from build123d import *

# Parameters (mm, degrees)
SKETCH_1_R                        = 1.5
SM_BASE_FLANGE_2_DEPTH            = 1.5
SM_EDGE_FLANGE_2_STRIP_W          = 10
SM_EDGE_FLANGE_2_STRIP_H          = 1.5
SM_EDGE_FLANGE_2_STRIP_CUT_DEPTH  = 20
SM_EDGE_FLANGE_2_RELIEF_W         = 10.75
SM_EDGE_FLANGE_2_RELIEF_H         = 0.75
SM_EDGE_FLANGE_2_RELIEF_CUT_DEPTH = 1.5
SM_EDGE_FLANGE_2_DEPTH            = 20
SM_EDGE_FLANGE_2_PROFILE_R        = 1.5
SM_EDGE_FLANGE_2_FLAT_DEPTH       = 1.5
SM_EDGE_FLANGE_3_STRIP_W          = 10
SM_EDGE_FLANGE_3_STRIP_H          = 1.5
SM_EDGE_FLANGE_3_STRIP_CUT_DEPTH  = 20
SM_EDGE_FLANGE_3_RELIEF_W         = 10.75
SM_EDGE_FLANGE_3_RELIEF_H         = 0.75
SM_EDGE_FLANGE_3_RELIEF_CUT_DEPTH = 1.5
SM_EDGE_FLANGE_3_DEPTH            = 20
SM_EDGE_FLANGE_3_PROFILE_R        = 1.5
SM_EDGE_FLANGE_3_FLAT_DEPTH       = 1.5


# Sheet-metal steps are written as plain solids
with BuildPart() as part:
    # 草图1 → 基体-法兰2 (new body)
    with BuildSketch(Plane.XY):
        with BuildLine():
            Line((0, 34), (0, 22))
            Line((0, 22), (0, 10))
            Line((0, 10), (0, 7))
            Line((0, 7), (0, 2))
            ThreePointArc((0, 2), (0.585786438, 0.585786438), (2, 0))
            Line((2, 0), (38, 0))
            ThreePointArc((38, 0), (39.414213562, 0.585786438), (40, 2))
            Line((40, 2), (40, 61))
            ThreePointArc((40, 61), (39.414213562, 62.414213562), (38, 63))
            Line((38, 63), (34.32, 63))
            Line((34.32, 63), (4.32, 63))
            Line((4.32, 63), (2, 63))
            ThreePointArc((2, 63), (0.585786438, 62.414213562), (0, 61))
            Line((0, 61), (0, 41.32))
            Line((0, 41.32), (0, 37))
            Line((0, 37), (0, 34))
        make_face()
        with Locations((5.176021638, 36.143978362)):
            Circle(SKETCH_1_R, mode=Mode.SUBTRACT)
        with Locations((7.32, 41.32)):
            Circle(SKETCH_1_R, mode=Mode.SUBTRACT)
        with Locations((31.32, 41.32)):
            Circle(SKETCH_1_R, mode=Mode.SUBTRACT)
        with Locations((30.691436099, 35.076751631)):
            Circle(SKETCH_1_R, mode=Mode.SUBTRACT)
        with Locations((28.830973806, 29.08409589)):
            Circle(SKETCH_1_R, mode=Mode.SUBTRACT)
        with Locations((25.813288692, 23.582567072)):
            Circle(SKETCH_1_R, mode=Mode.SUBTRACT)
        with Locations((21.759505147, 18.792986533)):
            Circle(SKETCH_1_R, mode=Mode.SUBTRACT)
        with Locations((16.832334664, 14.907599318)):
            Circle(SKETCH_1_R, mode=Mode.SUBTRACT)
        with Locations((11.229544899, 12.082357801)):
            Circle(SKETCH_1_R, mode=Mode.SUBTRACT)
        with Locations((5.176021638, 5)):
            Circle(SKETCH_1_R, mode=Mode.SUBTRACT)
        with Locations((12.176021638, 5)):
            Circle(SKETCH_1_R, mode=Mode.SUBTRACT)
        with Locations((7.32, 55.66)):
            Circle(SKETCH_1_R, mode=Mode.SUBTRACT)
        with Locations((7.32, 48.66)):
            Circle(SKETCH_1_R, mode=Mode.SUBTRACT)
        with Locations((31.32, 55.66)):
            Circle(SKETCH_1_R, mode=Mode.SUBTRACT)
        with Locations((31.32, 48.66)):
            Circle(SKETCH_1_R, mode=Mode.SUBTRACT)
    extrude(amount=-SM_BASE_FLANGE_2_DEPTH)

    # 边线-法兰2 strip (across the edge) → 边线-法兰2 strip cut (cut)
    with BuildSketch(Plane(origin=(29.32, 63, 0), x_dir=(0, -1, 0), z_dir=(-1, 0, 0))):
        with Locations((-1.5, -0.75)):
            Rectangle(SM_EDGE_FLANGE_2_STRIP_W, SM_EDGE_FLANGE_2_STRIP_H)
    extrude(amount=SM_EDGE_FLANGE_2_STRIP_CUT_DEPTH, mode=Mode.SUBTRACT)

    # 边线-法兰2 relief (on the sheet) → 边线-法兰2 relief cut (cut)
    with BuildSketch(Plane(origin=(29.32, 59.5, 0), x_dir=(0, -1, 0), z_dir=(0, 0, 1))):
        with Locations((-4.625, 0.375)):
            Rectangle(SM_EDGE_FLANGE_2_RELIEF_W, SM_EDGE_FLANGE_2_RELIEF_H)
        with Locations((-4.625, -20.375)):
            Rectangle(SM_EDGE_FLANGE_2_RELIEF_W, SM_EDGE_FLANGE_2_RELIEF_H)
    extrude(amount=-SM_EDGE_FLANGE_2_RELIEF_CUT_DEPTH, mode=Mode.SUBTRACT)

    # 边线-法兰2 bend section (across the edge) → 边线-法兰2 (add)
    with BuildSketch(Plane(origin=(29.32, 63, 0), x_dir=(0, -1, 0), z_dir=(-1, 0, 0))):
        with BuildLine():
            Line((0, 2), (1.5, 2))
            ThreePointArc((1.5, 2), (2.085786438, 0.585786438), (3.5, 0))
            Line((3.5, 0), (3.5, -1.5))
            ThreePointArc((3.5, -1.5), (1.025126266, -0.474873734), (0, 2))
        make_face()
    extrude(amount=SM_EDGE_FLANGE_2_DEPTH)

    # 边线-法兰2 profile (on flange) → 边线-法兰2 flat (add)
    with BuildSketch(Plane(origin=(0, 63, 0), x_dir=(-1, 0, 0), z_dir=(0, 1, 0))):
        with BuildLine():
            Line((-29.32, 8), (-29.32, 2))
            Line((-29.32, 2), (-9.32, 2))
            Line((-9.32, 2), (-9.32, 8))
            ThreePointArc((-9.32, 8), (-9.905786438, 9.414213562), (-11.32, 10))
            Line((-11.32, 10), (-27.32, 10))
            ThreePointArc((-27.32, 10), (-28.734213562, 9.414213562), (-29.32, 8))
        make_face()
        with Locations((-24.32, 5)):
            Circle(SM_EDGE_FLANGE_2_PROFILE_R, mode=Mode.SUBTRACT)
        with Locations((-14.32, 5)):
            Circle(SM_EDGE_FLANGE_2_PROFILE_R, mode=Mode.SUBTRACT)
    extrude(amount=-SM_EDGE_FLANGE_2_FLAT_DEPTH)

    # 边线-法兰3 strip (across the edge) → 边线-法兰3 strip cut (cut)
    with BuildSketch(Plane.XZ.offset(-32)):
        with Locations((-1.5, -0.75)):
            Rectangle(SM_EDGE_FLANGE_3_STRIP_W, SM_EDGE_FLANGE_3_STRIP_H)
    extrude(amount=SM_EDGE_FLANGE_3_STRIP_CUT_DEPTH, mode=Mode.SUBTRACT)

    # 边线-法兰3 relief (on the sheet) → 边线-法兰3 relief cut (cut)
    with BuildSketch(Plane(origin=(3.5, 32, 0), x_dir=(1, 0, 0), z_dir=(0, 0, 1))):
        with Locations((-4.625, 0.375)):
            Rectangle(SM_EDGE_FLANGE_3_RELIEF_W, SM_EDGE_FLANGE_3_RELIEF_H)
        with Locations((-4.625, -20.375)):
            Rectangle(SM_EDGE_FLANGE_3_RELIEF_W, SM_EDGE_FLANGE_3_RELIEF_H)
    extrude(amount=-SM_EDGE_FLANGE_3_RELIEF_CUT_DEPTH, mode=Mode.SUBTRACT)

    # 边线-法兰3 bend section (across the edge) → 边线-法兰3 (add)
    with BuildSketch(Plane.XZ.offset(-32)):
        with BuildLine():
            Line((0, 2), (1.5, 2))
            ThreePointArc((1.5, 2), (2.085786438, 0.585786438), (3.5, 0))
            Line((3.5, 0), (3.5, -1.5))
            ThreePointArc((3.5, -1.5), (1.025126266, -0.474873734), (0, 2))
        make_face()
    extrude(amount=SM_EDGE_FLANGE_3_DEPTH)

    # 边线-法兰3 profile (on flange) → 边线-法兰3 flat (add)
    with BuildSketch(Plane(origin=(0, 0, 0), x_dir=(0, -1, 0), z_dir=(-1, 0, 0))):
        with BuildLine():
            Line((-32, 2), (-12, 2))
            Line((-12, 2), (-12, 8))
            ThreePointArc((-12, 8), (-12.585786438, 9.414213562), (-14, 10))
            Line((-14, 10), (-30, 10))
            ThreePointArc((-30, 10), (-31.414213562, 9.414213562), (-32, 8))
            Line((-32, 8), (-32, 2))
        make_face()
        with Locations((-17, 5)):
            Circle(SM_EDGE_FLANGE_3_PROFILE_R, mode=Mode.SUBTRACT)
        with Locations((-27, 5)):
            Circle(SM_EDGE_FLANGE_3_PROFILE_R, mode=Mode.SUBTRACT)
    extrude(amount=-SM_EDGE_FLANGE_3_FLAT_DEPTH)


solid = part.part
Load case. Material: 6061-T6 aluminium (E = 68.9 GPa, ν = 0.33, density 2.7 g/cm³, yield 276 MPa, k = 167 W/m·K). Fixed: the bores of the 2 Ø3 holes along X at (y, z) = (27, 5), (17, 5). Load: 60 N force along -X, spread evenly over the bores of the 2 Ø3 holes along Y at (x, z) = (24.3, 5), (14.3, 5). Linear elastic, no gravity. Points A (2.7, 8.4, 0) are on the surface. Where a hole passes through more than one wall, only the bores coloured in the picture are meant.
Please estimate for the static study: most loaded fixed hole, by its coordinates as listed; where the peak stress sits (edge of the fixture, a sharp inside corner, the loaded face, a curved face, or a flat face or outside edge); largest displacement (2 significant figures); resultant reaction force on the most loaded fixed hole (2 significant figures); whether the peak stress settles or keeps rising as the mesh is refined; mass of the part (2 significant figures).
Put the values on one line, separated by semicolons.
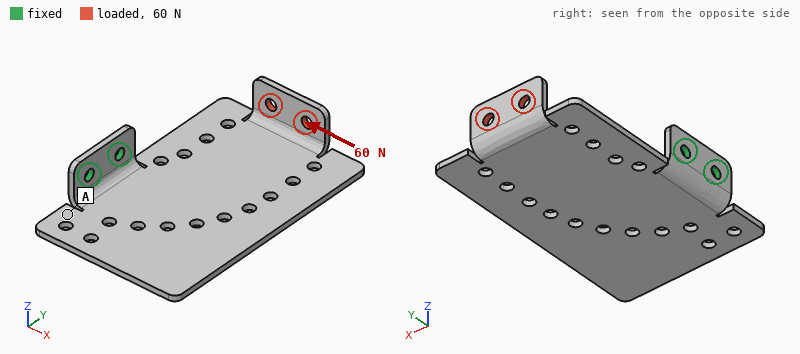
(27, 5); edge of the fixture; 0.50 mm; 230 N; keeps rising; 11 g
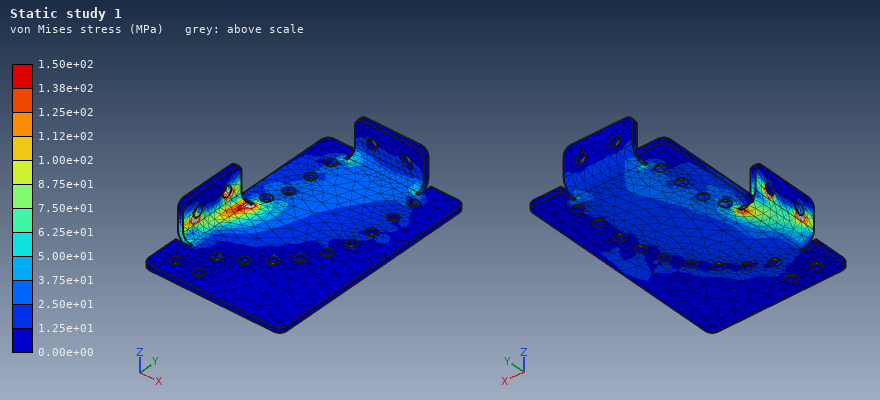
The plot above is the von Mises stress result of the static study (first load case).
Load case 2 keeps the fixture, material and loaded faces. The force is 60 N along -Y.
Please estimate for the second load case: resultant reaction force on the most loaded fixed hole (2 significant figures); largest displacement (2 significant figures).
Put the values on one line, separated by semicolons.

100 N; 0.76 mm
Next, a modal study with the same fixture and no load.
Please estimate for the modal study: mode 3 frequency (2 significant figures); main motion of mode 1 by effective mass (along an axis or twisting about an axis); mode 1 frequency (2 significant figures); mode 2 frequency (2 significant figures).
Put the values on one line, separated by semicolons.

1200 Hz; along Z; 370 Hz; 600 Hz
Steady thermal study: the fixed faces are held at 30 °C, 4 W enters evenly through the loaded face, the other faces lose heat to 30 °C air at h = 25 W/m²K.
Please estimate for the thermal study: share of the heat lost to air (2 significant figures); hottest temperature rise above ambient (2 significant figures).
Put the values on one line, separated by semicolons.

40 %; 28 K
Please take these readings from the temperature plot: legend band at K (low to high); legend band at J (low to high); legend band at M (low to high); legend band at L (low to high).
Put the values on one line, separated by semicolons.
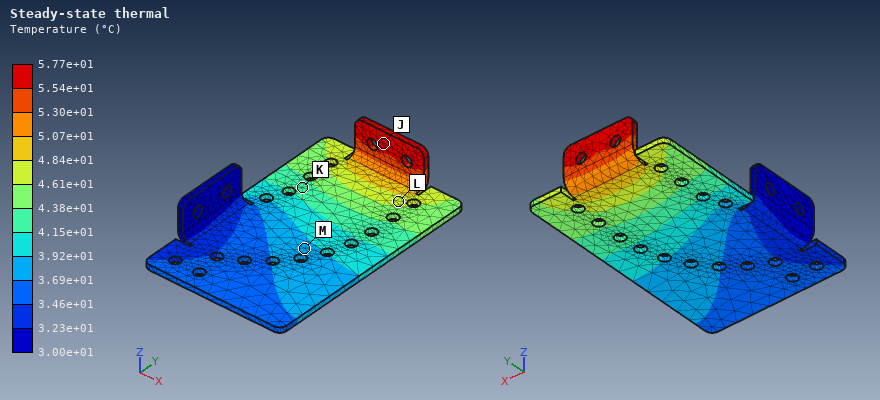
4.15e+01 to 4.38e+01 °C; 5.54e+01 to 5.77e+01 °C; 3.69e+01 to 3.92e+01 °C; 4.61e+01 to 4.84e+01 °C
